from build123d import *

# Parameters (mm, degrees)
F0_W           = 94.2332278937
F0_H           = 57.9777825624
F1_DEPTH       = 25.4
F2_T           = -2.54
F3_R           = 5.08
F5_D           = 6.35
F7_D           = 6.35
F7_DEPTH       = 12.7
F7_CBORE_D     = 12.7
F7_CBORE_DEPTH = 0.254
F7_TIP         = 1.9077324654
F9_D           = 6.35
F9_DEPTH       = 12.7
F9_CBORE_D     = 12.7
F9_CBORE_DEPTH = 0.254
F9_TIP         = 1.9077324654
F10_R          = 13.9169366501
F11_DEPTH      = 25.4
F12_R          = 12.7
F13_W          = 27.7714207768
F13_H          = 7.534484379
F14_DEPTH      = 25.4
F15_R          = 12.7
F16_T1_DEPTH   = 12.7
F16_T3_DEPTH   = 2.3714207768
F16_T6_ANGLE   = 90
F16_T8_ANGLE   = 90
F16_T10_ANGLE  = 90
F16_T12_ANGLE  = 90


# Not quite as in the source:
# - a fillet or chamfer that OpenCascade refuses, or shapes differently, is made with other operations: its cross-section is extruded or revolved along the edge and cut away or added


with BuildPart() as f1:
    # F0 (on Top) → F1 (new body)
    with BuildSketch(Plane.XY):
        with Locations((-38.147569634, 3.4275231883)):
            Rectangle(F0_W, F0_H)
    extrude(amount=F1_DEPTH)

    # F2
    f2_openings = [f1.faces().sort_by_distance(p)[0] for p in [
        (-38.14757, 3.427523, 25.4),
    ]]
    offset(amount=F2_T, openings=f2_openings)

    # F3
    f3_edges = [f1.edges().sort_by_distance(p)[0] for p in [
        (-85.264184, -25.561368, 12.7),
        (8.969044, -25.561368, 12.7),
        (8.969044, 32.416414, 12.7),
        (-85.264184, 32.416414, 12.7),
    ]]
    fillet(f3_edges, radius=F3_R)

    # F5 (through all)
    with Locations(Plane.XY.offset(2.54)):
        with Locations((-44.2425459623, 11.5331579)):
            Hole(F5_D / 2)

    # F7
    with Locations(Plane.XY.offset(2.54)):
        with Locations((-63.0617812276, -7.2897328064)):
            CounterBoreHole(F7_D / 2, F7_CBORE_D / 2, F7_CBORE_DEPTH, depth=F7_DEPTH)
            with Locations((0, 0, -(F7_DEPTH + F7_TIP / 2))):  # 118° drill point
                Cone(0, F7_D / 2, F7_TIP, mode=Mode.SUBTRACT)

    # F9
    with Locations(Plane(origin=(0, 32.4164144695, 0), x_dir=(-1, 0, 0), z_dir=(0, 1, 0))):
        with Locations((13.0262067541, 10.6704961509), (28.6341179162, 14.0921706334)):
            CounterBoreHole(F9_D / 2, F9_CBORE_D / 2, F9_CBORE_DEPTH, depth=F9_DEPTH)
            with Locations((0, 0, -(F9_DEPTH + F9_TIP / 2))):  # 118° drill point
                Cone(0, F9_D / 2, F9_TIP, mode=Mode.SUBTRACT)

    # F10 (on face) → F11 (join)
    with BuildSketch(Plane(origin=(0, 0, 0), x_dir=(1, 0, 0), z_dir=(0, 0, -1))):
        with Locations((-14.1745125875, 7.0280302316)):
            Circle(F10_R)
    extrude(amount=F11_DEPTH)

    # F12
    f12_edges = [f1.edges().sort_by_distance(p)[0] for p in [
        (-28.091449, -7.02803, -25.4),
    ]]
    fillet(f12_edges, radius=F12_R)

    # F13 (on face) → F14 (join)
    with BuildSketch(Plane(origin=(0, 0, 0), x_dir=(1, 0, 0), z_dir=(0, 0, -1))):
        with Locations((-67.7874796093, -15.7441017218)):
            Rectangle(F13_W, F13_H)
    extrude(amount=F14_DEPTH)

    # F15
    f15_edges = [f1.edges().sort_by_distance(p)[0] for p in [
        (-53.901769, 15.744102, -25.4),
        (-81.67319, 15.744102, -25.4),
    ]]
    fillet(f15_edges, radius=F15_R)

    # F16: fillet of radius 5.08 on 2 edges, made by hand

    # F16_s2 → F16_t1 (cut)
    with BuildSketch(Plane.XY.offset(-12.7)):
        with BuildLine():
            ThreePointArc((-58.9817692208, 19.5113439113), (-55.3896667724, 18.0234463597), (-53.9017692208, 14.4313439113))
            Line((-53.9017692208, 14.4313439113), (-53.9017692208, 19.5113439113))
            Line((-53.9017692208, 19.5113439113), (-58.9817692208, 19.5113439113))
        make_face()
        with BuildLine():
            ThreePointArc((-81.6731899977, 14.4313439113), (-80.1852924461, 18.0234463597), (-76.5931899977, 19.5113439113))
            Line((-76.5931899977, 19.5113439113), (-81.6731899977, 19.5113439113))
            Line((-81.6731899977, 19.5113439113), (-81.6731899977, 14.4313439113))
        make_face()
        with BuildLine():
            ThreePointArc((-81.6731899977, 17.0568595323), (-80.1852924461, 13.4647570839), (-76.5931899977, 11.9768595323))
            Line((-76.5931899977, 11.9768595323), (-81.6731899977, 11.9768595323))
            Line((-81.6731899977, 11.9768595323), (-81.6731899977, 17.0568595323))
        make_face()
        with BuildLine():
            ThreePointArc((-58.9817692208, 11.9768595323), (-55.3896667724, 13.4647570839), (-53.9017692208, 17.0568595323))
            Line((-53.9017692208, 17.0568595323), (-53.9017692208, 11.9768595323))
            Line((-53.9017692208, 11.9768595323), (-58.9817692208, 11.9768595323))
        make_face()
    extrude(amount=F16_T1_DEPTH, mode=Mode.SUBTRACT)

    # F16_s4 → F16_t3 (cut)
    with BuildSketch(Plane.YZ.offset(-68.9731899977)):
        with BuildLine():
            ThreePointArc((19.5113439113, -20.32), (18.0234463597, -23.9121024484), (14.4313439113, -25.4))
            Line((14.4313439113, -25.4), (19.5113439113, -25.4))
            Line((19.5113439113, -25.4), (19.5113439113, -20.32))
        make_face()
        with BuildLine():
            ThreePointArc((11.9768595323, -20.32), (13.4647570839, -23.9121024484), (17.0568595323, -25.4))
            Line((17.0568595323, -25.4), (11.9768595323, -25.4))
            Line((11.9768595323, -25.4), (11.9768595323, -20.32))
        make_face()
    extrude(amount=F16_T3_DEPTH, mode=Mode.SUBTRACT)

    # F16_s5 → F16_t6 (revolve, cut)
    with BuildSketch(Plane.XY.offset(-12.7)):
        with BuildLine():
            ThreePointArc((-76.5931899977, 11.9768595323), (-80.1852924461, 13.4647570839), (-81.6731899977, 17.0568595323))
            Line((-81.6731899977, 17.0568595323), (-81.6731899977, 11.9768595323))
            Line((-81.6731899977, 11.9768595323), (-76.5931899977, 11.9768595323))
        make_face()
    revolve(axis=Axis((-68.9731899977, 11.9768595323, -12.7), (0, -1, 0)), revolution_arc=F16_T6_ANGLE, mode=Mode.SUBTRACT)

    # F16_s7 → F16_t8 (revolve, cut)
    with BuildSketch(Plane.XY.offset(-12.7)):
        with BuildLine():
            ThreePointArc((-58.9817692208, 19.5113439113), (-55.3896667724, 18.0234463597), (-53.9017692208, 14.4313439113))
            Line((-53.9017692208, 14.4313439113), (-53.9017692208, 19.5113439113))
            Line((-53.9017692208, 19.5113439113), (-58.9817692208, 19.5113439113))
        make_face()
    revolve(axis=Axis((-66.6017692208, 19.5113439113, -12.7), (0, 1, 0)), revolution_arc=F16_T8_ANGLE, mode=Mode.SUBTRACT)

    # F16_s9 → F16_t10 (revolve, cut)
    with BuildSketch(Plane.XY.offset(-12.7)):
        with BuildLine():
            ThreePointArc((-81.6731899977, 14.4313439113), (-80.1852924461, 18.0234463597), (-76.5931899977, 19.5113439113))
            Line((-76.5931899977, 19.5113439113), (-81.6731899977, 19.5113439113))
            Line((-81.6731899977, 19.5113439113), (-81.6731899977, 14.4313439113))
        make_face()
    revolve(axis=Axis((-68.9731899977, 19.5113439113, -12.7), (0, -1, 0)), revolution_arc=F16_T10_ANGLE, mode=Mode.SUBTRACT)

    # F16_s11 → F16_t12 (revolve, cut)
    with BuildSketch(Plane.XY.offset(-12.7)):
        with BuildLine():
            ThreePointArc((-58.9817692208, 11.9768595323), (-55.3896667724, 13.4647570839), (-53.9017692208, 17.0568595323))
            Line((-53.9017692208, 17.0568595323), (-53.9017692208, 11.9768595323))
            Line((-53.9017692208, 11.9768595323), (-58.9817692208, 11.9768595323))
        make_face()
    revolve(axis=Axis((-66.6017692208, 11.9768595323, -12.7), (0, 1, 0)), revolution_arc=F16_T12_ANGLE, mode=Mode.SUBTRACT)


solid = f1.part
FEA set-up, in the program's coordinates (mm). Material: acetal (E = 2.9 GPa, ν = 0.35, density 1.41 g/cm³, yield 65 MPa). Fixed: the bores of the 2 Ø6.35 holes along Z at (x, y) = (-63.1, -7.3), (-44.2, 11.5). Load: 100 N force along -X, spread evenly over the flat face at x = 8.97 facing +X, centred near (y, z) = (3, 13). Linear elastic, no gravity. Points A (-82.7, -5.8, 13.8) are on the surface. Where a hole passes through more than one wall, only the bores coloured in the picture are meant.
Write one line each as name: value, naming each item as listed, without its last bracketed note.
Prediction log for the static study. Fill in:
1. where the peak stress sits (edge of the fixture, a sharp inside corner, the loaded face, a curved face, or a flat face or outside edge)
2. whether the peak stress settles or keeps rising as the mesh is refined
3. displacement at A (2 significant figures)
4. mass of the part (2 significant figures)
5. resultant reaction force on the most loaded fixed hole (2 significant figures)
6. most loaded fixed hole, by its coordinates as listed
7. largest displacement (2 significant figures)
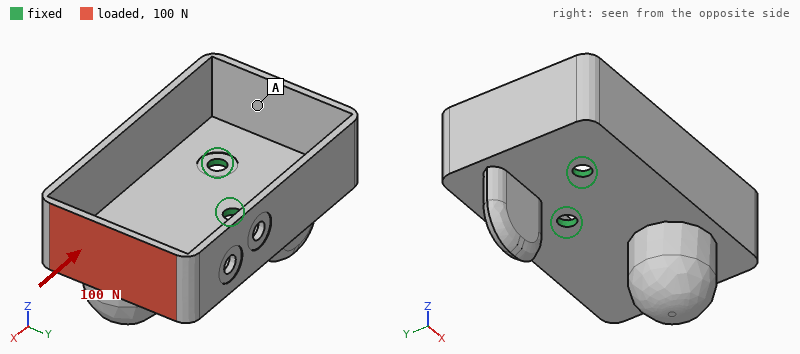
where the peak stress sits: edge of the fixture
whether the peak stress settles or keeps rising as the mesh is refined: keeps rising
displacement at A: 0.33 mm
mass of the part: 66 g
resultant reaction force on the most loaded fixed hole: 62 N
most loaded fixed hole, by its coordinates as listed: (-44.2, 11.5)
largest displacement: 1.2 mm
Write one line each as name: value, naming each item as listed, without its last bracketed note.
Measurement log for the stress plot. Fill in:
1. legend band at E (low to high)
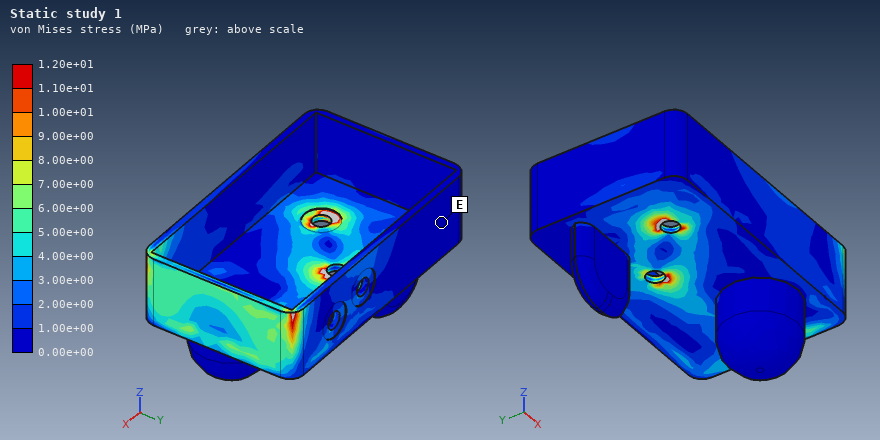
legend band at E: 0.00e+00 to 1.00e+00 MPa
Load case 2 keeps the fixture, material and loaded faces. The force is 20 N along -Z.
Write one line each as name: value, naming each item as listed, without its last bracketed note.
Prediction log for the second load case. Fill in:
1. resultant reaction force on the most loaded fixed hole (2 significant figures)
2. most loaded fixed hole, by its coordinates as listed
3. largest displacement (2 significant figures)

resultant reaction force on the most loaded fixed hole: 33 N
most loaded fixed hole, by its coordinates as listed: (-44.2, 11.5)
largest displacement: 1.3 mm
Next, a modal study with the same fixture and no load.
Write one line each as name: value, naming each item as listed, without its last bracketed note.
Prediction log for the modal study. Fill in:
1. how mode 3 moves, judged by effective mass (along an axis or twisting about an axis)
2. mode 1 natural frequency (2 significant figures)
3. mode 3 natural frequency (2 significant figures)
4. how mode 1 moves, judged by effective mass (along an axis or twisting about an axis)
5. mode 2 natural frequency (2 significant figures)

how mode 3 moves, judged by effective mass: along Z
mode 1 natural frequency: 140 Hz
mode 3 natural frequency: 380 Hz
how mode 1 moves, judged by effective mass: along Z
mode 2 natural frequency: 310 Hz
